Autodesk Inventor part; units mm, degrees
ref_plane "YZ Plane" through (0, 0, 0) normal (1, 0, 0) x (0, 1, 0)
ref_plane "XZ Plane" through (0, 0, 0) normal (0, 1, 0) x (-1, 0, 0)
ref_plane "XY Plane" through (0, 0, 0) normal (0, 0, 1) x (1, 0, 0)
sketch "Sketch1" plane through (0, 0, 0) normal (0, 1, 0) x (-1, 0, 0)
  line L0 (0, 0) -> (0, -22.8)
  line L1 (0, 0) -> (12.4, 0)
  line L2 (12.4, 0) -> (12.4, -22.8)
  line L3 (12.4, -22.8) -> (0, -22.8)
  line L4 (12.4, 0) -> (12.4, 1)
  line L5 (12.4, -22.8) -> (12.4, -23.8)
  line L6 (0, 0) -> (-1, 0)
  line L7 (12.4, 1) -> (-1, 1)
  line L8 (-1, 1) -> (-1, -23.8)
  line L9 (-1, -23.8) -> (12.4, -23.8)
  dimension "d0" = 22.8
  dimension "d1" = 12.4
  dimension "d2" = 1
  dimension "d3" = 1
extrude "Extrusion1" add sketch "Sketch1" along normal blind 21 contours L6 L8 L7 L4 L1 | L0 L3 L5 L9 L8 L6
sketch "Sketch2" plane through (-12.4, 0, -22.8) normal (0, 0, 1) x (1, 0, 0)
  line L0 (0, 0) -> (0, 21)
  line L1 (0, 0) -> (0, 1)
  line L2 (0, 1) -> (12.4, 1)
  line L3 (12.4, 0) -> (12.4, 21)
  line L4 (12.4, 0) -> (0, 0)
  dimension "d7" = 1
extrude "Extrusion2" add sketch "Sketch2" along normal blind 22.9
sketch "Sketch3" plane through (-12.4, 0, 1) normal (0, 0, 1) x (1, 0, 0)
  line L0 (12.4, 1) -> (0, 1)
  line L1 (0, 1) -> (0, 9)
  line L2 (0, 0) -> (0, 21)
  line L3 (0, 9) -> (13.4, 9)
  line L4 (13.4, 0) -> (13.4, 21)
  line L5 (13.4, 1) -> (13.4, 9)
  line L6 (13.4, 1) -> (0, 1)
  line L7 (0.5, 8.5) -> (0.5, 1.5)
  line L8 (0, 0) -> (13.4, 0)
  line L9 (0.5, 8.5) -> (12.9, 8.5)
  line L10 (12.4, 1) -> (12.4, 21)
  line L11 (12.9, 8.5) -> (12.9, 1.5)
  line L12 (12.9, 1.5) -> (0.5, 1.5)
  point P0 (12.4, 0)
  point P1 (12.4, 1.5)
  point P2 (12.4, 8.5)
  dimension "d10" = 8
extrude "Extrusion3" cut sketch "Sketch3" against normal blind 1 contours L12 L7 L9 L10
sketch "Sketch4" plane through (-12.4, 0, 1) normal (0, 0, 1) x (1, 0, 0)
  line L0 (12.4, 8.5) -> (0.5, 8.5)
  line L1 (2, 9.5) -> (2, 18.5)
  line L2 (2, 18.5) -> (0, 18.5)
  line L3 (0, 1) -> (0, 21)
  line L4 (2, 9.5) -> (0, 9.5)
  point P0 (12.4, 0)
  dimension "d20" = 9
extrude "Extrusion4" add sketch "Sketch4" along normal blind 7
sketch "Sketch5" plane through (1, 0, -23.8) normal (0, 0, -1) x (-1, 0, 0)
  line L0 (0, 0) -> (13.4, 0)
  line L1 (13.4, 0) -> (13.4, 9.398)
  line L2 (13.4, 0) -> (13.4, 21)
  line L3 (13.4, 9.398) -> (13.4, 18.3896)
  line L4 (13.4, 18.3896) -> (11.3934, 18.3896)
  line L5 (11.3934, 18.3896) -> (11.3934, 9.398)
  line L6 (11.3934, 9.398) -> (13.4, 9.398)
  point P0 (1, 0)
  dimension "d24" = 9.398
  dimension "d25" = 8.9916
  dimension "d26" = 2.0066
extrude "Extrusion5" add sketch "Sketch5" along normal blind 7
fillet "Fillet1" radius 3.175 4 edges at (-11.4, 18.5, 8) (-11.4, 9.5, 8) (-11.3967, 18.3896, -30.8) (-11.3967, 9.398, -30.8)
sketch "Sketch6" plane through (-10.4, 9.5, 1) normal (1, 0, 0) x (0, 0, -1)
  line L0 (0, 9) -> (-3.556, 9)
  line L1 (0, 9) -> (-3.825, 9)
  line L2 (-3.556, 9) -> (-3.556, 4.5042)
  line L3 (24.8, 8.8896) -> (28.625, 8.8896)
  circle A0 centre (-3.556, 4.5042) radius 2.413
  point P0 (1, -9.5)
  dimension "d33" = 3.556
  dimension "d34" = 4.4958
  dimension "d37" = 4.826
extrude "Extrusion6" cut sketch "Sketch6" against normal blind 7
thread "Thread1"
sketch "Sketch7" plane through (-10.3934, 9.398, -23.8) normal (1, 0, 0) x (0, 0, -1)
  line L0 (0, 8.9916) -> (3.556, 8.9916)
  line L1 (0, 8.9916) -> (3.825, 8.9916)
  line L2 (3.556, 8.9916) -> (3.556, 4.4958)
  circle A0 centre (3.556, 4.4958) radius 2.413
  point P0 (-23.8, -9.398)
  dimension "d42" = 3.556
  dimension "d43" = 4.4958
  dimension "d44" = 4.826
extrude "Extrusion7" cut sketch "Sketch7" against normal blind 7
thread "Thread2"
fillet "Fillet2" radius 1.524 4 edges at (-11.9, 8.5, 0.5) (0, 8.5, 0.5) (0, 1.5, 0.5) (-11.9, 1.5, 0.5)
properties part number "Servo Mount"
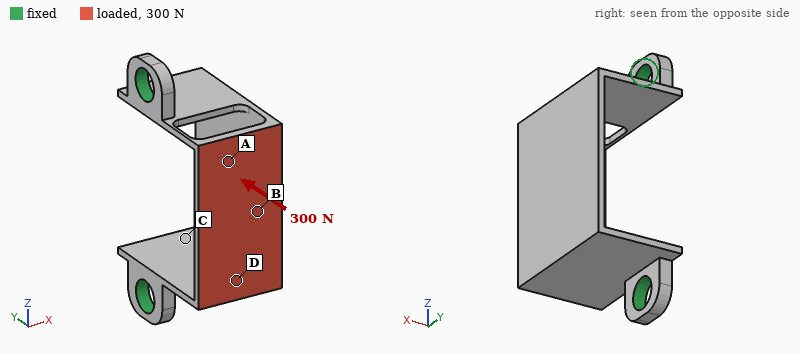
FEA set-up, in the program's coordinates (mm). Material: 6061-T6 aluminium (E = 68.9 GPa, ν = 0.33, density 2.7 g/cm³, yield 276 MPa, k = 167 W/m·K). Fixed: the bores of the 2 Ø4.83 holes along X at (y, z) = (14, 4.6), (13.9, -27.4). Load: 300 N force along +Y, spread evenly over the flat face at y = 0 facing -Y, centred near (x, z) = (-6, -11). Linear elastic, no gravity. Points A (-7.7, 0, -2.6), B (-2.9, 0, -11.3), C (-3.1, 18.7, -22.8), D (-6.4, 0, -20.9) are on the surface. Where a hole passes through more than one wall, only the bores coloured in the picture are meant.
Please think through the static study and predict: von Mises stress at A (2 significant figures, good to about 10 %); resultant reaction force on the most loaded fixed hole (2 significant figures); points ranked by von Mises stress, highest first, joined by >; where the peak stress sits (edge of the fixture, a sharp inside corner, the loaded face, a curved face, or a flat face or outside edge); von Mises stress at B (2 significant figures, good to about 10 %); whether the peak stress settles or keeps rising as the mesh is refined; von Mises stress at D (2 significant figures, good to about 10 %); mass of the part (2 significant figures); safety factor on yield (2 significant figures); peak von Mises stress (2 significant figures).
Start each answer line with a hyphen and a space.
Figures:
- 110 MPa
- 150 N
- A > D > B > C
- a curved face
- 34 MPa
- settles
- 82 MPa
- 3.8 g
- 0.44
- 620 MPa
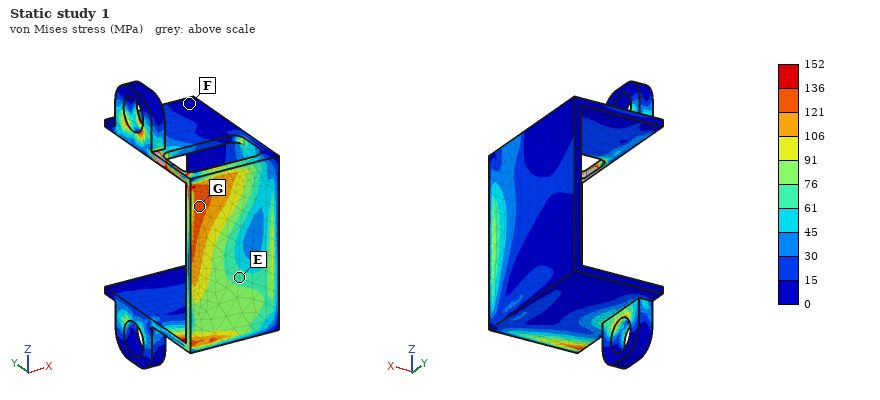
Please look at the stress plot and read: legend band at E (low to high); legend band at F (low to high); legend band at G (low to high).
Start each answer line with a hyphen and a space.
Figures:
- 61 to 76 MPa
- 0 to 15 MPa
- 121 to 136 MPa
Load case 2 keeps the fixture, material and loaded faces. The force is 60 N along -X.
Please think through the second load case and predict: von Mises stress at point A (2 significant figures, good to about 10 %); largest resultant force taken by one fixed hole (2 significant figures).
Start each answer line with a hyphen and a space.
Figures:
- 16 MPa
- 32 N
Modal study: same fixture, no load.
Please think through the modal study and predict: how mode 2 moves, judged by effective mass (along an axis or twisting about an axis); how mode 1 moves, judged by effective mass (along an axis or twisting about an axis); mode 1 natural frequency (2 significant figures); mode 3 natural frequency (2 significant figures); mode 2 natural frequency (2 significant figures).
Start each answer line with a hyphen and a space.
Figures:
- along X
- along Z
- 3300 Hz
- 6000 Hz
- 4500 Hz
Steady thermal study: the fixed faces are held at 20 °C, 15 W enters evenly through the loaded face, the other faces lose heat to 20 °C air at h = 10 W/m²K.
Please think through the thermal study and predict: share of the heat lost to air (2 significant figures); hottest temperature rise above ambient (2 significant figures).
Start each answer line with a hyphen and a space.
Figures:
- 5.8 %
- 73 K
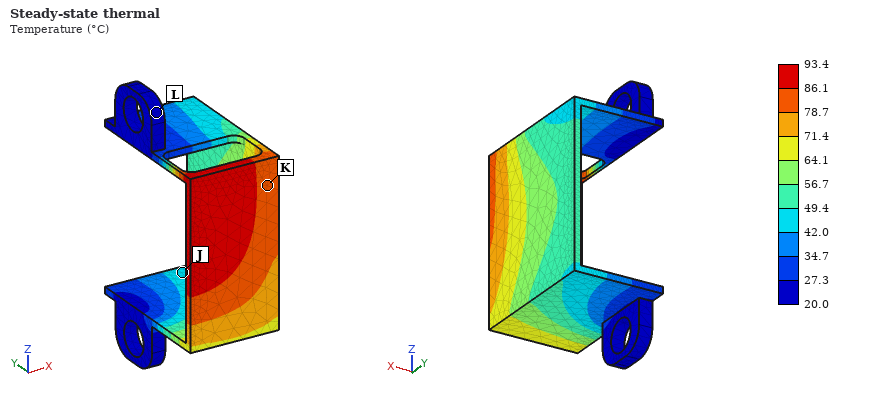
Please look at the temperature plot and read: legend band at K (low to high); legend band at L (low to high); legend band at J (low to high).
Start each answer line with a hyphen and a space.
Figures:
- 78.7 to 86.1 °C
- 20.0 to 27.3 °C
- 42.0 to 49.4 °C
